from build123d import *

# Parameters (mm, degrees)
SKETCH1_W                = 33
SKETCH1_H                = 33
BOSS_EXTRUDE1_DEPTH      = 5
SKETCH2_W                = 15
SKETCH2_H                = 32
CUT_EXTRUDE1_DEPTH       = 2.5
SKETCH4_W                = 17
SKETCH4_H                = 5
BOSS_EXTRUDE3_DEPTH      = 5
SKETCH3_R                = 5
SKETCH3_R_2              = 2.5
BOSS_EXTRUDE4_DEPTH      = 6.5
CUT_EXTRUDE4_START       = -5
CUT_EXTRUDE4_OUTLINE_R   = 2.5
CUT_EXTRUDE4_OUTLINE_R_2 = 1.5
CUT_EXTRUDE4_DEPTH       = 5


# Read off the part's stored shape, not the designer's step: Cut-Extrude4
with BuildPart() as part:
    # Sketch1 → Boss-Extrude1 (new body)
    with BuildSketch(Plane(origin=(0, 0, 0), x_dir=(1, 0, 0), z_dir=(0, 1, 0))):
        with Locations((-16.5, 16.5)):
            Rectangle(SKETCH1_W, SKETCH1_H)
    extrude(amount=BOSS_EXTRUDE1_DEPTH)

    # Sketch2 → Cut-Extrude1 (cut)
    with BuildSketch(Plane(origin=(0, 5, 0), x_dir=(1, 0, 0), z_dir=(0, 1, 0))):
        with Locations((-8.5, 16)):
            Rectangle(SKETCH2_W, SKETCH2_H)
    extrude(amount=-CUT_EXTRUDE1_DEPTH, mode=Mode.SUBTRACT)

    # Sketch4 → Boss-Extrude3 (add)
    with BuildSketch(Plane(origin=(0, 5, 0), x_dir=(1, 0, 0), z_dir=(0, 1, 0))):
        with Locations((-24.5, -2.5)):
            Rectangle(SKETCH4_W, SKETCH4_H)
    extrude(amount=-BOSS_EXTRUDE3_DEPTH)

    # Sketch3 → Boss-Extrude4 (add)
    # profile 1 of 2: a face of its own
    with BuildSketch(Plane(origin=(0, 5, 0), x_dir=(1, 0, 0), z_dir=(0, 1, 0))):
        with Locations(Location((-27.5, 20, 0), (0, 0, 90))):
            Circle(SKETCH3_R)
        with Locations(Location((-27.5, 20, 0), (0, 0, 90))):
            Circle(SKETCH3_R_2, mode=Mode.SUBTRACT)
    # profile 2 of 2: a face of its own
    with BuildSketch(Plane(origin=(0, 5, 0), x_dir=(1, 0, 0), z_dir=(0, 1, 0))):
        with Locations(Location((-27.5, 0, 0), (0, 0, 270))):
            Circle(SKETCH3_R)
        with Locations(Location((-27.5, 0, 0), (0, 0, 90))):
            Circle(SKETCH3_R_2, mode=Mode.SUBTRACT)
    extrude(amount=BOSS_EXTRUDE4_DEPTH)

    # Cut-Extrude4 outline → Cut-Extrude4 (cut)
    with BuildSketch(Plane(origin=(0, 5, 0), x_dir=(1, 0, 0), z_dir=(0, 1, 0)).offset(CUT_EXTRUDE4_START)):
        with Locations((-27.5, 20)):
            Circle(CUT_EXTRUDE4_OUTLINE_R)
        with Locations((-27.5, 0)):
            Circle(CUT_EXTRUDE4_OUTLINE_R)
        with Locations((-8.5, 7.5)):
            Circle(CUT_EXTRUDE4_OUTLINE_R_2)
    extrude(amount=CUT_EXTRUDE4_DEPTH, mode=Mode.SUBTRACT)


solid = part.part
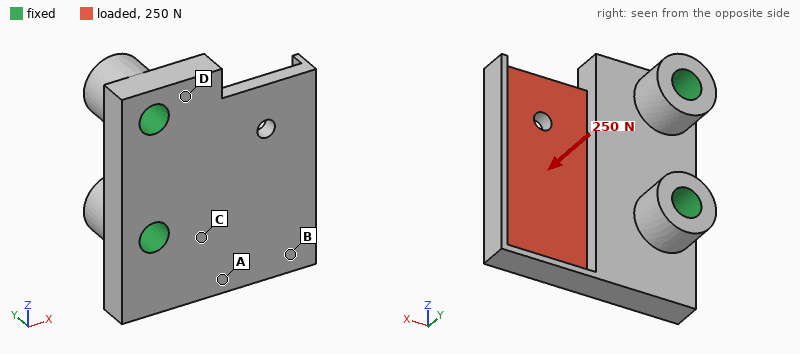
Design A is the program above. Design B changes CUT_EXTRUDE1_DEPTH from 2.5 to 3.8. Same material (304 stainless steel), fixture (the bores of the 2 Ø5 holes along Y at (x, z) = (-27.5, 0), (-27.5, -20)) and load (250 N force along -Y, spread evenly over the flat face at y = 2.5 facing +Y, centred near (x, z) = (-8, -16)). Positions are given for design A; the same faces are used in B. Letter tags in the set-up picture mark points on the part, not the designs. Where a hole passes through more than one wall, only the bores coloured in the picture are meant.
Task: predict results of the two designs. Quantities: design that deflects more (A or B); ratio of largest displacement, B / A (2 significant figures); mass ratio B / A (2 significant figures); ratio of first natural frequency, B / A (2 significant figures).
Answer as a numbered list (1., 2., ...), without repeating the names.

1. B
2. 5.7
3. 0.88
4. 0.59
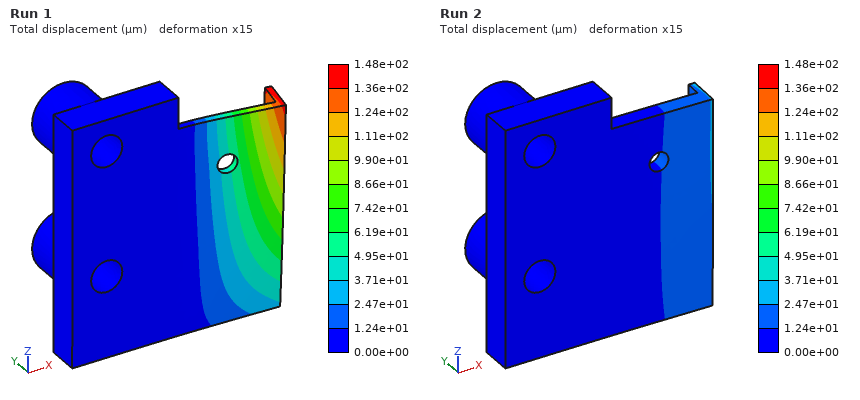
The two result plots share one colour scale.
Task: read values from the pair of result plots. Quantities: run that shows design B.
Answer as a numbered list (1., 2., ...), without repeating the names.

1. Run 1
